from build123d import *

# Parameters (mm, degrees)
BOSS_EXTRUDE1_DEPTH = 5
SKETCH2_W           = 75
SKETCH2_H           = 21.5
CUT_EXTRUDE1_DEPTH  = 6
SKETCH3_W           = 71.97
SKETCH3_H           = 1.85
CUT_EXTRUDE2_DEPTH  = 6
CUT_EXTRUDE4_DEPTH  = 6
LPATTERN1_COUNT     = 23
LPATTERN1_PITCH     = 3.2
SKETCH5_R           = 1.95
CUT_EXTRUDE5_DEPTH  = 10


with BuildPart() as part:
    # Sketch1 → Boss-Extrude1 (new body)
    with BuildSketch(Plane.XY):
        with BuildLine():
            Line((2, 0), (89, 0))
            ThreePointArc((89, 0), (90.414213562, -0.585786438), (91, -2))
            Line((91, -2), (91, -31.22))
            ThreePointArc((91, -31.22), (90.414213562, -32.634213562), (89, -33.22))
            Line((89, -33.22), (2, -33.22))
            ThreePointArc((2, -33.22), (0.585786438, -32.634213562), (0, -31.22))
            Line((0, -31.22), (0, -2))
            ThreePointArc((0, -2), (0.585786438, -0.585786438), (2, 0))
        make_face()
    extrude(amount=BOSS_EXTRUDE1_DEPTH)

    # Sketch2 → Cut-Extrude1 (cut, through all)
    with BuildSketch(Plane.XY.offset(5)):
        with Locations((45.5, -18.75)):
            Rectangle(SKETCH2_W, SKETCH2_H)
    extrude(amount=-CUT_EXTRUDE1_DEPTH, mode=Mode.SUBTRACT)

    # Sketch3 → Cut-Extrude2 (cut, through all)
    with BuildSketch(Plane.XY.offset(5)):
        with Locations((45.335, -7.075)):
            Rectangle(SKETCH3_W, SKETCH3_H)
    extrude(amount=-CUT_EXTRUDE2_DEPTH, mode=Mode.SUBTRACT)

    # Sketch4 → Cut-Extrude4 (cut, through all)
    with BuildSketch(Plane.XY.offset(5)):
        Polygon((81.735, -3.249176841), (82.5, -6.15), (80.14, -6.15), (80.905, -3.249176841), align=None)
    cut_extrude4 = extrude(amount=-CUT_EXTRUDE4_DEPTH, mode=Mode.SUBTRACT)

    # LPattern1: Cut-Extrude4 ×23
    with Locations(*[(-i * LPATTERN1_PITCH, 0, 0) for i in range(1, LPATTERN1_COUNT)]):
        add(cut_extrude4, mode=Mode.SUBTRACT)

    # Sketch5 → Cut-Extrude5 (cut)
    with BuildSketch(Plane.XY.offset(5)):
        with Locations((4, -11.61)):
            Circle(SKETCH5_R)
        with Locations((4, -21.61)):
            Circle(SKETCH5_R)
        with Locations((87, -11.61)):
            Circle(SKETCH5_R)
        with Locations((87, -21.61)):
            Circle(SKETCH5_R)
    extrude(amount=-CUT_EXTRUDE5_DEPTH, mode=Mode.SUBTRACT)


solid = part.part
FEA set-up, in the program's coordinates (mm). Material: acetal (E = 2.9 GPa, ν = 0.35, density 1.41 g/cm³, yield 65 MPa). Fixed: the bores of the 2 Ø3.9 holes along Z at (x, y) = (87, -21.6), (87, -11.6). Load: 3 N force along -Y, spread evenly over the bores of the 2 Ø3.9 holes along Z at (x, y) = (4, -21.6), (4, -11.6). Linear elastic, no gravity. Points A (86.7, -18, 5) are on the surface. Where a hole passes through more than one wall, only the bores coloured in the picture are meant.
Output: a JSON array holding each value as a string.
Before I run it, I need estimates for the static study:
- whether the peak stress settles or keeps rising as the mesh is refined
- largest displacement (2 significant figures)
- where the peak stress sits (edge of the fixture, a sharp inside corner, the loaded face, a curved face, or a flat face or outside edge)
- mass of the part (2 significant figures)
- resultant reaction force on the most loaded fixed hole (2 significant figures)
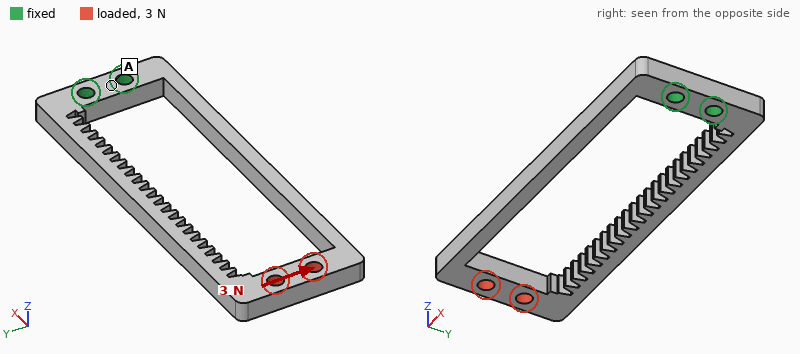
["keeps rising", "1.1 mm", "a sharp inside corner", "7.9 g", "8.6 N"]
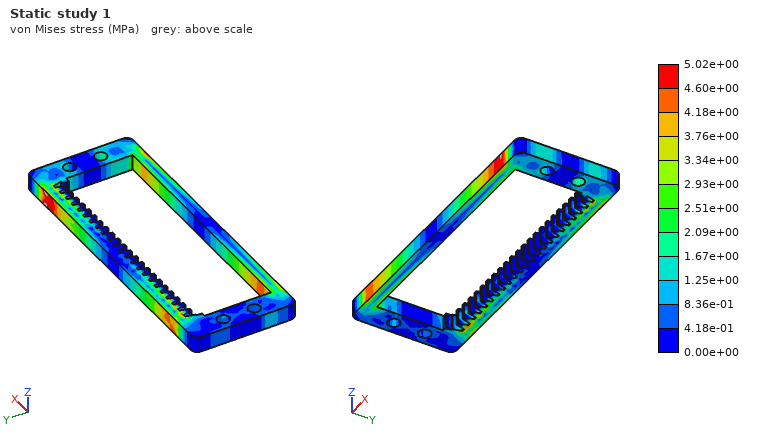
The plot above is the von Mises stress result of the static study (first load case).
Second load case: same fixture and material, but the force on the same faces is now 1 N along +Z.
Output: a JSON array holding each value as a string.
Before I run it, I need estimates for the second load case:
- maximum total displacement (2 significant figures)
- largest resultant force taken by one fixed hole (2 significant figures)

["1.0 mm", "0.50 N"]
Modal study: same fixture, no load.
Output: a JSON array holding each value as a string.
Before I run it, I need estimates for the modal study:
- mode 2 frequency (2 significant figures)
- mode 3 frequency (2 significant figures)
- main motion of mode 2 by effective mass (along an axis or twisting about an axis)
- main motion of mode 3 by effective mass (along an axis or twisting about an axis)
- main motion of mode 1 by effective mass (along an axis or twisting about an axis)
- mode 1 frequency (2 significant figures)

["140 Hz", "320 Hz", "along Y", "twisting about X", "along Z", "100 Hz"]
